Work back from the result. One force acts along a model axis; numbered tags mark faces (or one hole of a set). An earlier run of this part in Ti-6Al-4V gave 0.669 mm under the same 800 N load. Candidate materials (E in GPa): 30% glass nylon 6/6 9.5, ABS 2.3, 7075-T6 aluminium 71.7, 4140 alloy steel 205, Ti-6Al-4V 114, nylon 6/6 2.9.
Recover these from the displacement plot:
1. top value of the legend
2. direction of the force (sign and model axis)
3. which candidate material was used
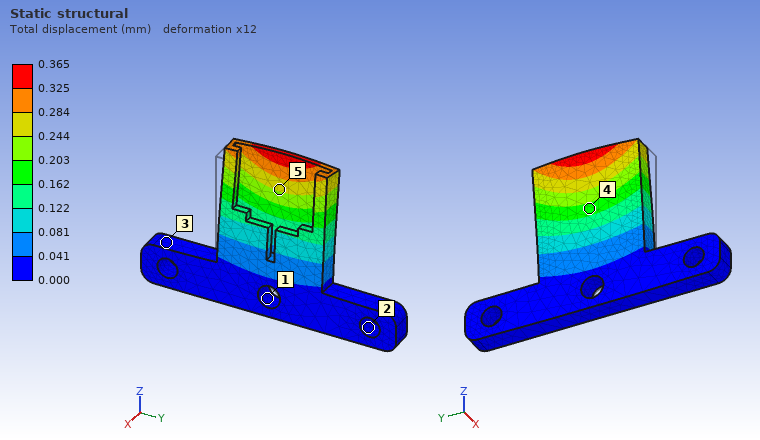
0.365 mm
-X
4140 alloy steel
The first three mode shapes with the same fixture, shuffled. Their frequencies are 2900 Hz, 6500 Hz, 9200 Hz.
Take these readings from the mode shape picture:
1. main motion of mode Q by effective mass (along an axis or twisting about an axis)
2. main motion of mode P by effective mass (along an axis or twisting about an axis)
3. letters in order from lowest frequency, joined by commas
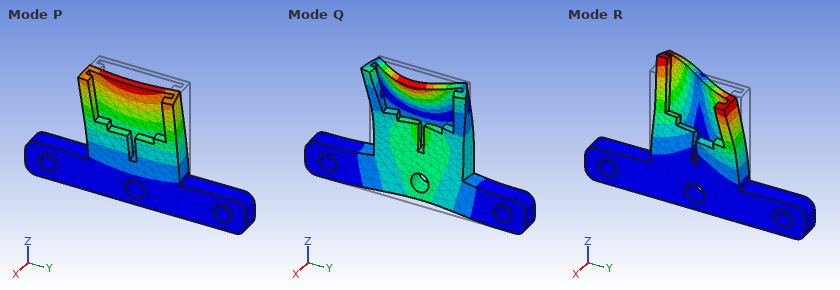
along X
along X
P, R, Q
